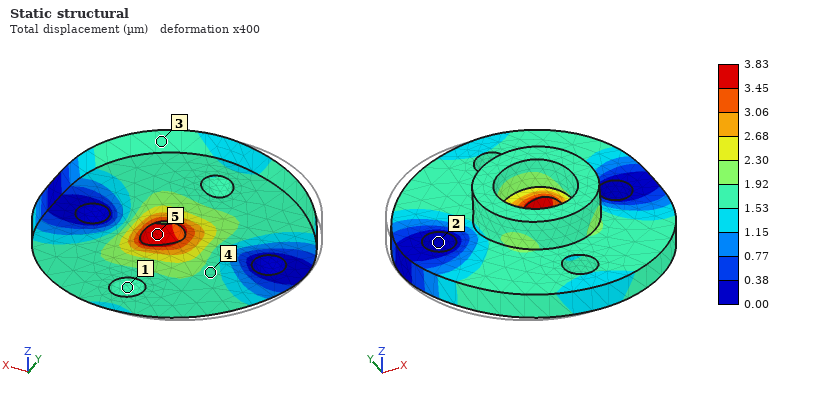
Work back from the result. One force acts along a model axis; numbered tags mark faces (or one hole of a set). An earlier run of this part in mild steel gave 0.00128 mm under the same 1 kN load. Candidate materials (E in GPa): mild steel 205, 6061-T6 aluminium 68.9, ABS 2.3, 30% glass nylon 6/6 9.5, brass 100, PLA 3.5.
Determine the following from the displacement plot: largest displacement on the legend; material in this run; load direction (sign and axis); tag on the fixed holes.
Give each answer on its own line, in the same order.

3.83 µm
6061-T6 aluminium
+X
2
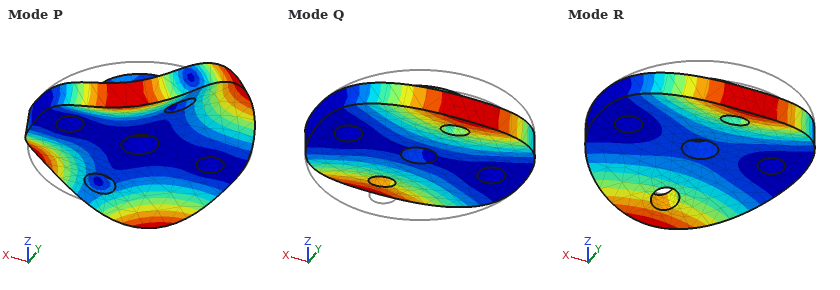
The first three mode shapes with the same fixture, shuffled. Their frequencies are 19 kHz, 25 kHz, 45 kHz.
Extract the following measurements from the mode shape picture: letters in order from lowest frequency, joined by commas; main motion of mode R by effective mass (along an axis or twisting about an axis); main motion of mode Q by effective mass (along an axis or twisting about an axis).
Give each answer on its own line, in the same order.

Q, R, P
along Z
twisting about X
